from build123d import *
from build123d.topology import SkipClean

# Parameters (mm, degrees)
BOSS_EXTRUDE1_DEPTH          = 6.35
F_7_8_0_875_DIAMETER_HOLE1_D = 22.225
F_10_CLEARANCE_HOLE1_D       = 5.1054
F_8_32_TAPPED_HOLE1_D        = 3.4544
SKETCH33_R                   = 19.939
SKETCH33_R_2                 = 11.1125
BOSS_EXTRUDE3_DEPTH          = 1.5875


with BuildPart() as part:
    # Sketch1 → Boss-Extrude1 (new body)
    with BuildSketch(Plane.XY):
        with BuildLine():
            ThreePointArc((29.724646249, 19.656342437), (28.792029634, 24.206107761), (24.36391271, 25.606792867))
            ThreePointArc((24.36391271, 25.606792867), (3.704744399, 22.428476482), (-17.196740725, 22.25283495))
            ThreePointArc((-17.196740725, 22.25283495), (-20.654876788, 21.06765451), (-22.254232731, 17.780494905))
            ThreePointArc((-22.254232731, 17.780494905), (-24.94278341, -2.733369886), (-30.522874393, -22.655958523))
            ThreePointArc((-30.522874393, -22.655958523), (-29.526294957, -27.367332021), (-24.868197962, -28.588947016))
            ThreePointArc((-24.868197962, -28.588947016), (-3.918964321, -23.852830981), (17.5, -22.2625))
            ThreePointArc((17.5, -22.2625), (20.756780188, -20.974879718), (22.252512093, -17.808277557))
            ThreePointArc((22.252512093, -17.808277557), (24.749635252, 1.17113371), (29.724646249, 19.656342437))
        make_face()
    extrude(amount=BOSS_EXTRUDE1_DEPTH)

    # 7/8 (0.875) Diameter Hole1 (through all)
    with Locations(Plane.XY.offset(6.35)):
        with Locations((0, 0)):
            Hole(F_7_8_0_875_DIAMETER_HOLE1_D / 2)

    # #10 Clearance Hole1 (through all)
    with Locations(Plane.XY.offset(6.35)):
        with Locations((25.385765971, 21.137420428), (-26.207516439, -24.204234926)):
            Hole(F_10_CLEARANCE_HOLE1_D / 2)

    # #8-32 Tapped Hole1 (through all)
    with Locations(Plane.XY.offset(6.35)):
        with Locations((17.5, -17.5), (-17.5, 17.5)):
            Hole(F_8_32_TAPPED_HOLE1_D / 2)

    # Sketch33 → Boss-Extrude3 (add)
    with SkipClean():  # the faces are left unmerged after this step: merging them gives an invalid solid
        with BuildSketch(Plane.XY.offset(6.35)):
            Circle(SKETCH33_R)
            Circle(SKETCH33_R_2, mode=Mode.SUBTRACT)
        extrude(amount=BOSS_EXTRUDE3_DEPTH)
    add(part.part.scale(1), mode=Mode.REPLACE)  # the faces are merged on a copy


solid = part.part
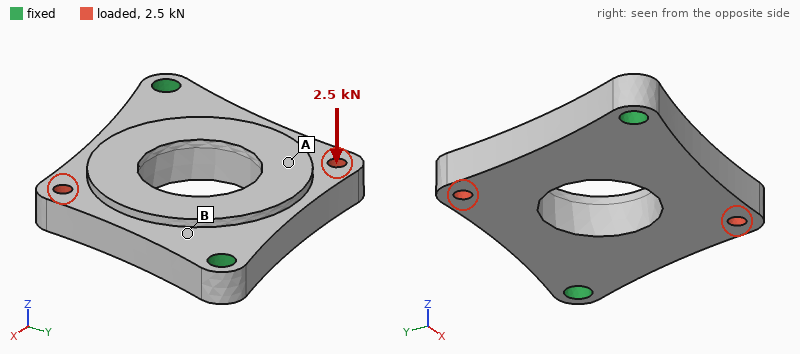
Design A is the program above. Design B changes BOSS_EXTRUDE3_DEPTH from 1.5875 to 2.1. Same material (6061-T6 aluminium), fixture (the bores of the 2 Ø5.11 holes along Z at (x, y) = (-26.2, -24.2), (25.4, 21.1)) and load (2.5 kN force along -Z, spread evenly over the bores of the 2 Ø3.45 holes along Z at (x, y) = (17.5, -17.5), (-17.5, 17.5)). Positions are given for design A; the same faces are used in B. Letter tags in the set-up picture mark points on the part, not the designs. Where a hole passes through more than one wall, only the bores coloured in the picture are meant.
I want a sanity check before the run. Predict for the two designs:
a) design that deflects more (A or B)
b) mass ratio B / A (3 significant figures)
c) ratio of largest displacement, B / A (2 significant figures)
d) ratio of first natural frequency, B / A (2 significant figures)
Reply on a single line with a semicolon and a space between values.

A; 1.03; 0.92; 1.00
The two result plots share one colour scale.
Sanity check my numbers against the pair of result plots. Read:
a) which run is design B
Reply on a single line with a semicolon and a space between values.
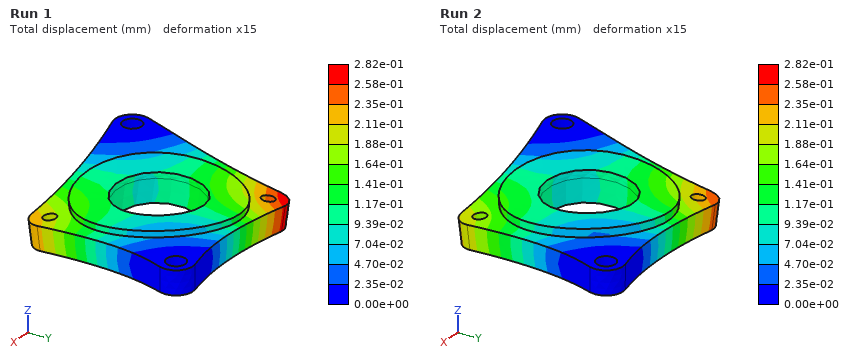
Run 2
